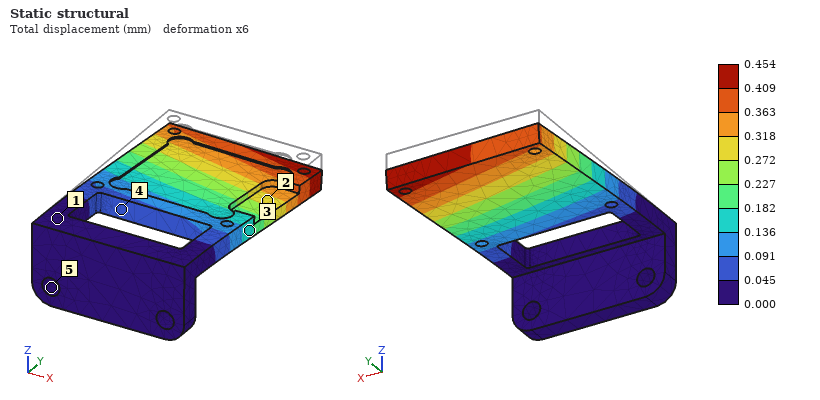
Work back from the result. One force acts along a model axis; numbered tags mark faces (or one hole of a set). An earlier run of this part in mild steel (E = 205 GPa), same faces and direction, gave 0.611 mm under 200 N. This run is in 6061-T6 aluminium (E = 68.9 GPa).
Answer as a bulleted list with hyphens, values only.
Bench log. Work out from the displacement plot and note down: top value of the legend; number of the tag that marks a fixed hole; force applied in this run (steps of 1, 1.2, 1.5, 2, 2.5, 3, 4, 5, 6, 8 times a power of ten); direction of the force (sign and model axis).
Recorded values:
- 0.454 mm
- 5
- 50 N
- -Z
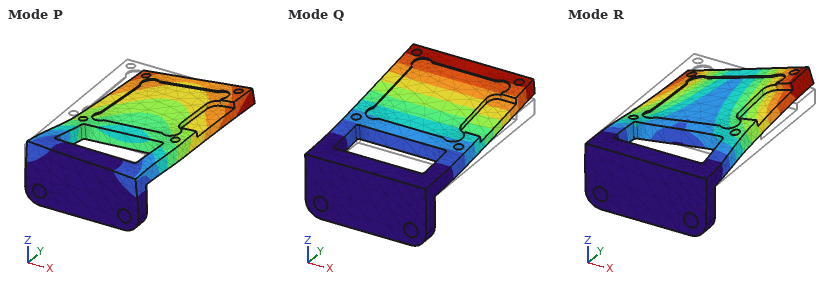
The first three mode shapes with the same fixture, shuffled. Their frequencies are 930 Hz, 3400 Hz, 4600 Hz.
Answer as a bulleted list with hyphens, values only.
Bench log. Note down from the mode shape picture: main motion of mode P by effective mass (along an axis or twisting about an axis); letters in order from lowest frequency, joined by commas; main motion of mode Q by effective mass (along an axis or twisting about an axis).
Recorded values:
- along X
- Q, P, R
- along Z
